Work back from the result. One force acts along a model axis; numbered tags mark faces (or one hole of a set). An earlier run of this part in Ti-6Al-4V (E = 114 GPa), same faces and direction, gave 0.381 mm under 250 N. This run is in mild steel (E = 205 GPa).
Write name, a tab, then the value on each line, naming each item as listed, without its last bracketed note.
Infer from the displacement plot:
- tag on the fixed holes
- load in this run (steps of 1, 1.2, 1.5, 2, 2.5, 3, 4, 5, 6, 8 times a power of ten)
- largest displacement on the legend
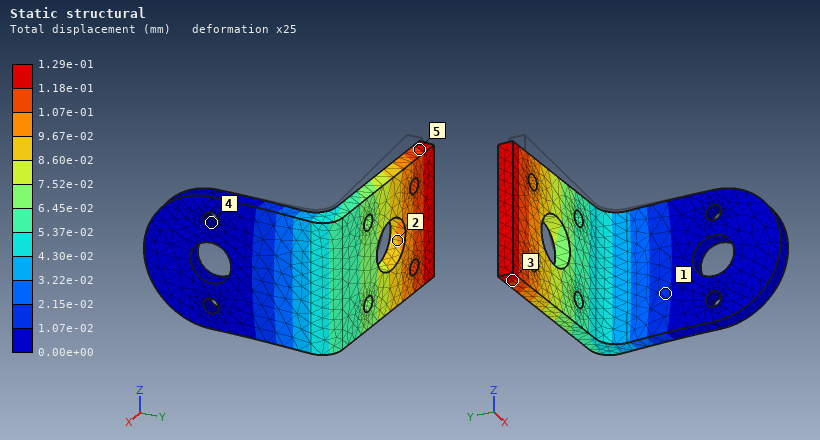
tag on the fixed holes	4
load in this run	150 N
largest displacement on the legend	1.29e-01 mm
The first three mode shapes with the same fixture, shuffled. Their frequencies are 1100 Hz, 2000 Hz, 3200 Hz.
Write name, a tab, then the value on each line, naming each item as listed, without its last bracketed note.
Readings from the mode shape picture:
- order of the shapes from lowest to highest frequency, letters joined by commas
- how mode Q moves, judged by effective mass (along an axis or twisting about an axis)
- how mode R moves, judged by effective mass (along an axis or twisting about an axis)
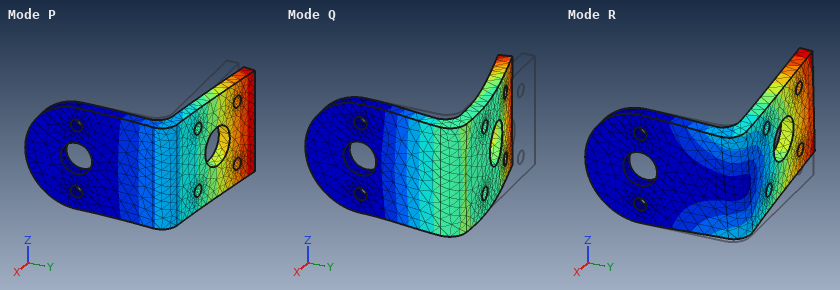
order of the shapes from lowest to highest frequency, letters joined by commas	P, R, Q
how mode Q moves, judged by effective mass	along X
how mode R moves, judged by effective mass	along Z
